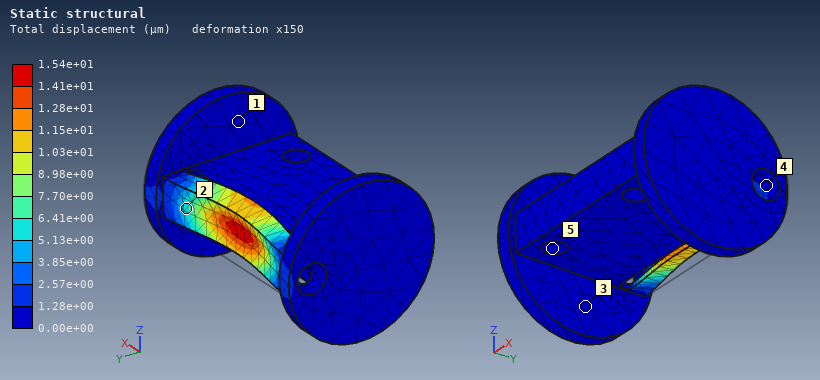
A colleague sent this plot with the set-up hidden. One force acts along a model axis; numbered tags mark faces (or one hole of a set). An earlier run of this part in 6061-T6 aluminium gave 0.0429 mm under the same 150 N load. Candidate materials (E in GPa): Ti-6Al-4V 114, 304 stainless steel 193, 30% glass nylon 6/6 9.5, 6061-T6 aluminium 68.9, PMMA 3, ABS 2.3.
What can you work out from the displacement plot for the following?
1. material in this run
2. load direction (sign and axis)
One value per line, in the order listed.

304 stainless steel
-Y
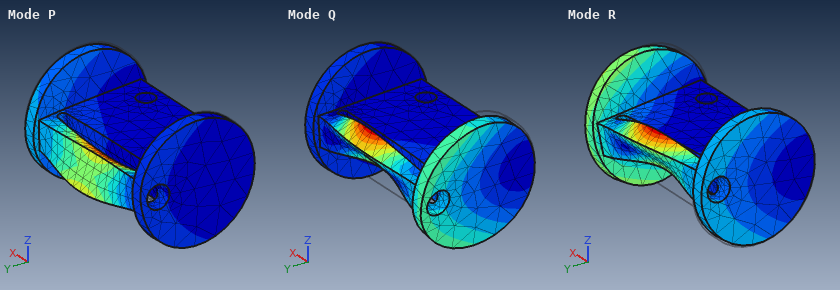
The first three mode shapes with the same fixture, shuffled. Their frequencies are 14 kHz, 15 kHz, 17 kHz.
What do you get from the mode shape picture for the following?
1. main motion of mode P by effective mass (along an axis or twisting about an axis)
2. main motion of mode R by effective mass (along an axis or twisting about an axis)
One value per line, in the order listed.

along Z
twisting about Y
